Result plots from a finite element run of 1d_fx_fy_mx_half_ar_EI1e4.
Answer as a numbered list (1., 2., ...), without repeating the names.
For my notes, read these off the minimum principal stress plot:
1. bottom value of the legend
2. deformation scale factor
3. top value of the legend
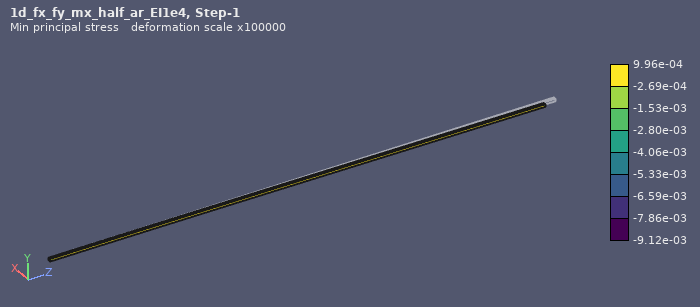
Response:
1. -9.12e-03
2. 100000
3. 9.96e-04
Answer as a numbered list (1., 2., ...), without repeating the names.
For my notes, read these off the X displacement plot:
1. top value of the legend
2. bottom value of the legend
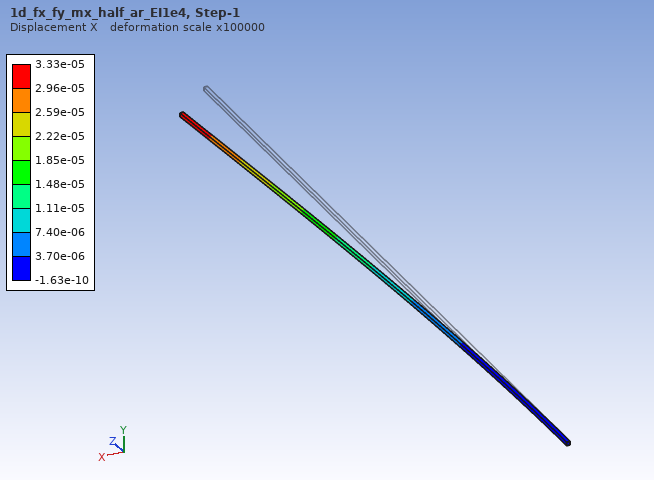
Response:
1. 3.33e-05
2. -1.63e-10
